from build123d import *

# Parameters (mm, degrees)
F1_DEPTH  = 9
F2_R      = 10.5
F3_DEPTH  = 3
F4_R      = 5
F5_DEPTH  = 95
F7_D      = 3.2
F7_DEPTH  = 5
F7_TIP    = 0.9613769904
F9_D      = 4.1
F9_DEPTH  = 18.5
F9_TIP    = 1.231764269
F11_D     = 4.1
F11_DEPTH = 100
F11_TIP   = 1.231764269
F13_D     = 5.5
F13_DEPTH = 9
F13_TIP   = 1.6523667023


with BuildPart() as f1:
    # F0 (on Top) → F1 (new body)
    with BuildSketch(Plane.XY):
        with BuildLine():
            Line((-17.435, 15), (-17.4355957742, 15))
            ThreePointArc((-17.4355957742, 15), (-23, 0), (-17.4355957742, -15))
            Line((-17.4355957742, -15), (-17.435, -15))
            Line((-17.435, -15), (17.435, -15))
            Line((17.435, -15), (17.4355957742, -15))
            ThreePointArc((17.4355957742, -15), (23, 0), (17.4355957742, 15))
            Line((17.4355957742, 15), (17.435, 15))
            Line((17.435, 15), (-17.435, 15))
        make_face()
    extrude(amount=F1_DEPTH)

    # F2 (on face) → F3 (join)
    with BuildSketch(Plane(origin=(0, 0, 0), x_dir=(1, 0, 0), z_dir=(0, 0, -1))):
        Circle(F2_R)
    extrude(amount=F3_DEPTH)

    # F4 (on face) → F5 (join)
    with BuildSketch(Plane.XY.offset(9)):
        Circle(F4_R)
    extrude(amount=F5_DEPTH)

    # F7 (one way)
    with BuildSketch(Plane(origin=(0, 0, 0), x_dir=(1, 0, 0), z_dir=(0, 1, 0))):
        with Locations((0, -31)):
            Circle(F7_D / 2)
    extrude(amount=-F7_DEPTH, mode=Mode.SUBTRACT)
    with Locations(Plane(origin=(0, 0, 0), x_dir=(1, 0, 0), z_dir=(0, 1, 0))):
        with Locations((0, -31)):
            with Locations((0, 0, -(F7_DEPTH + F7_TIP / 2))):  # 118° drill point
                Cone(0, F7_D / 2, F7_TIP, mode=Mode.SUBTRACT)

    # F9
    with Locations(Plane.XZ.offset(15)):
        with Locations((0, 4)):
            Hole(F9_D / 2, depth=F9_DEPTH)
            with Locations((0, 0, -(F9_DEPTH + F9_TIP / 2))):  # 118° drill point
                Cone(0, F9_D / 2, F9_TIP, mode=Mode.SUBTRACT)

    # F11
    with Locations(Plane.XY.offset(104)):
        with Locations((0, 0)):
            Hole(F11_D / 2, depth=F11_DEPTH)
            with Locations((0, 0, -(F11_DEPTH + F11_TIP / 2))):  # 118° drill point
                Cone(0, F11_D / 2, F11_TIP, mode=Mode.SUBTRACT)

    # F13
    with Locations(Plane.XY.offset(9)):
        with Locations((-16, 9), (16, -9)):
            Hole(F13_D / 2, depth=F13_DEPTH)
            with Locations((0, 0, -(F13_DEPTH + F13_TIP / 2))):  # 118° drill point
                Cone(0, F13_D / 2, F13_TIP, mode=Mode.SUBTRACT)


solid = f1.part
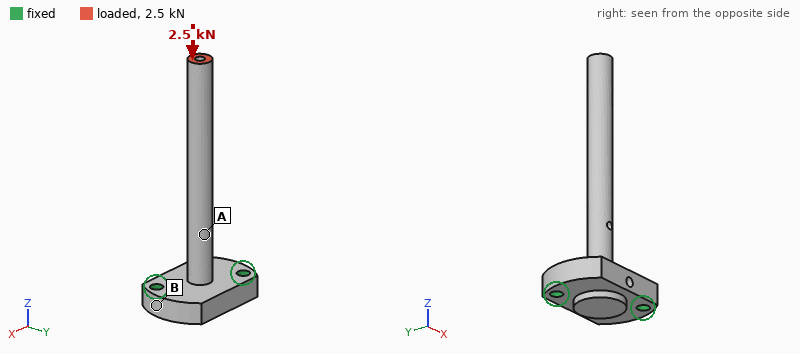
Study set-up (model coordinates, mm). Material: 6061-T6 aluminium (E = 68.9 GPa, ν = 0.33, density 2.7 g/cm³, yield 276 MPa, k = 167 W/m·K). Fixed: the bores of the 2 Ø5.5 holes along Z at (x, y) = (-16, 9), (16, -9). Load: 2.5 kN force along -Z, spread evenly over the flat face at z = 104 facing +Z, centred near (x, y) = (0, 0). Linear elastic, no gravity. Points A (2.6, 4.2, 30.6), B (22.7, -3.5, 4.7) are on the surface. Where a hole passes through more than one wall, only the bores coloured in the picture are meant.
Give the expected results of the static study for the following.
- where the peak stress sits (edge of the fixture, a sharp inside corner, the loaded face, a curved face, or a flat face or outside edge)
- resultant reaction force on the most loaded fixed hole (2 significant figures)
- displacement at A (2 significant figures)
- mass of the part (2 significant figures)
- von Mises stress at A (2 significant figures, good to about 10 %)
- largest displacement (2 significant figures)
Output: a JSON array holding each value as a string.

["a curved face", "1.3 kN", "20 µm", "49 g", "34 MPa", "71 µm"]
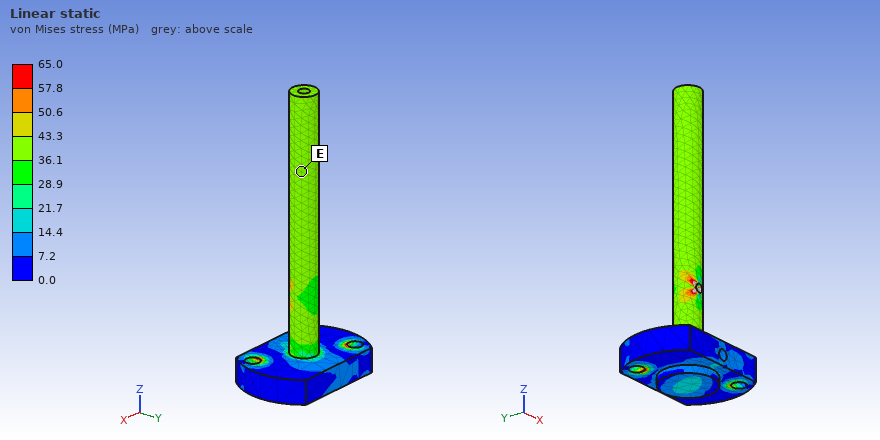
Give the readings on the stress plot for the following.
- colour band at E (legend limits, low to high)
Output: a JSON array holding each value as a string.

["36.1 to 43.3 MPa"]
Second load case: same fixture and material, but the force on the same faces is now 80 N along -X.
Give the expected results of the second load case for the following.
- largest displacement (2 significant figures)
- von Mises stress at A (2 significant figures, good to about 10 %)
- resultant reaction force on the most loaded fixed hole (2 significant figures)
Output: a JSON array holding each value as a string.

["0.78 mm", "33 MPa", "260 N"]
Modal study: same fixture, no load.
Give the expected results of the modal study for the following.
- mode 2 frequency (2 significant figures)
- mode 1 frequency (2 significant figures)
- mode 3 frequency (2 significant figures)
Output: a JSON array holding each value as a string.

["790 Hz", "760 Hz", "4600 Hz"]
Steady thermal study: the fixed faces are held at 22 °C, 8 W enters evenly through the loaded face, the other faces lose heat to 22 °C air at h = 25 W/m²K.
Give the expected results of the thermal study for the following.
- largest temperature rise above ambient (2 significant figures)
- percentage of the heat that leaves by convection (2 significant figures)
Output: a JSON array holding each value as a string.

["56 K", "36 %"]
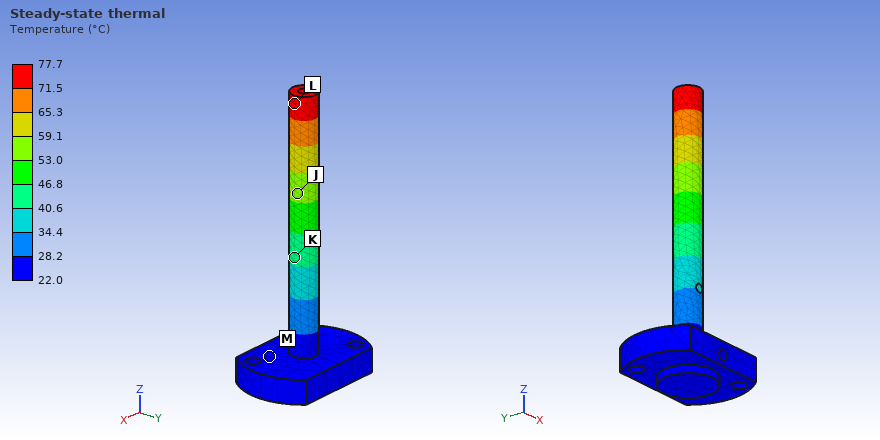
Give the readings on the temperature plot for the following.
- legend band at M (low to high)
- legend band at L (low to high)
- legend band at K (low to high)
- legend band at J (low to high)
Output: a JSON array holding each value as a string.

["22.0 to 28.2 °C", "71.5 to 77.7 °C", "40.6 to 46.8 °C", "53.0 to 59.1 °C"]
